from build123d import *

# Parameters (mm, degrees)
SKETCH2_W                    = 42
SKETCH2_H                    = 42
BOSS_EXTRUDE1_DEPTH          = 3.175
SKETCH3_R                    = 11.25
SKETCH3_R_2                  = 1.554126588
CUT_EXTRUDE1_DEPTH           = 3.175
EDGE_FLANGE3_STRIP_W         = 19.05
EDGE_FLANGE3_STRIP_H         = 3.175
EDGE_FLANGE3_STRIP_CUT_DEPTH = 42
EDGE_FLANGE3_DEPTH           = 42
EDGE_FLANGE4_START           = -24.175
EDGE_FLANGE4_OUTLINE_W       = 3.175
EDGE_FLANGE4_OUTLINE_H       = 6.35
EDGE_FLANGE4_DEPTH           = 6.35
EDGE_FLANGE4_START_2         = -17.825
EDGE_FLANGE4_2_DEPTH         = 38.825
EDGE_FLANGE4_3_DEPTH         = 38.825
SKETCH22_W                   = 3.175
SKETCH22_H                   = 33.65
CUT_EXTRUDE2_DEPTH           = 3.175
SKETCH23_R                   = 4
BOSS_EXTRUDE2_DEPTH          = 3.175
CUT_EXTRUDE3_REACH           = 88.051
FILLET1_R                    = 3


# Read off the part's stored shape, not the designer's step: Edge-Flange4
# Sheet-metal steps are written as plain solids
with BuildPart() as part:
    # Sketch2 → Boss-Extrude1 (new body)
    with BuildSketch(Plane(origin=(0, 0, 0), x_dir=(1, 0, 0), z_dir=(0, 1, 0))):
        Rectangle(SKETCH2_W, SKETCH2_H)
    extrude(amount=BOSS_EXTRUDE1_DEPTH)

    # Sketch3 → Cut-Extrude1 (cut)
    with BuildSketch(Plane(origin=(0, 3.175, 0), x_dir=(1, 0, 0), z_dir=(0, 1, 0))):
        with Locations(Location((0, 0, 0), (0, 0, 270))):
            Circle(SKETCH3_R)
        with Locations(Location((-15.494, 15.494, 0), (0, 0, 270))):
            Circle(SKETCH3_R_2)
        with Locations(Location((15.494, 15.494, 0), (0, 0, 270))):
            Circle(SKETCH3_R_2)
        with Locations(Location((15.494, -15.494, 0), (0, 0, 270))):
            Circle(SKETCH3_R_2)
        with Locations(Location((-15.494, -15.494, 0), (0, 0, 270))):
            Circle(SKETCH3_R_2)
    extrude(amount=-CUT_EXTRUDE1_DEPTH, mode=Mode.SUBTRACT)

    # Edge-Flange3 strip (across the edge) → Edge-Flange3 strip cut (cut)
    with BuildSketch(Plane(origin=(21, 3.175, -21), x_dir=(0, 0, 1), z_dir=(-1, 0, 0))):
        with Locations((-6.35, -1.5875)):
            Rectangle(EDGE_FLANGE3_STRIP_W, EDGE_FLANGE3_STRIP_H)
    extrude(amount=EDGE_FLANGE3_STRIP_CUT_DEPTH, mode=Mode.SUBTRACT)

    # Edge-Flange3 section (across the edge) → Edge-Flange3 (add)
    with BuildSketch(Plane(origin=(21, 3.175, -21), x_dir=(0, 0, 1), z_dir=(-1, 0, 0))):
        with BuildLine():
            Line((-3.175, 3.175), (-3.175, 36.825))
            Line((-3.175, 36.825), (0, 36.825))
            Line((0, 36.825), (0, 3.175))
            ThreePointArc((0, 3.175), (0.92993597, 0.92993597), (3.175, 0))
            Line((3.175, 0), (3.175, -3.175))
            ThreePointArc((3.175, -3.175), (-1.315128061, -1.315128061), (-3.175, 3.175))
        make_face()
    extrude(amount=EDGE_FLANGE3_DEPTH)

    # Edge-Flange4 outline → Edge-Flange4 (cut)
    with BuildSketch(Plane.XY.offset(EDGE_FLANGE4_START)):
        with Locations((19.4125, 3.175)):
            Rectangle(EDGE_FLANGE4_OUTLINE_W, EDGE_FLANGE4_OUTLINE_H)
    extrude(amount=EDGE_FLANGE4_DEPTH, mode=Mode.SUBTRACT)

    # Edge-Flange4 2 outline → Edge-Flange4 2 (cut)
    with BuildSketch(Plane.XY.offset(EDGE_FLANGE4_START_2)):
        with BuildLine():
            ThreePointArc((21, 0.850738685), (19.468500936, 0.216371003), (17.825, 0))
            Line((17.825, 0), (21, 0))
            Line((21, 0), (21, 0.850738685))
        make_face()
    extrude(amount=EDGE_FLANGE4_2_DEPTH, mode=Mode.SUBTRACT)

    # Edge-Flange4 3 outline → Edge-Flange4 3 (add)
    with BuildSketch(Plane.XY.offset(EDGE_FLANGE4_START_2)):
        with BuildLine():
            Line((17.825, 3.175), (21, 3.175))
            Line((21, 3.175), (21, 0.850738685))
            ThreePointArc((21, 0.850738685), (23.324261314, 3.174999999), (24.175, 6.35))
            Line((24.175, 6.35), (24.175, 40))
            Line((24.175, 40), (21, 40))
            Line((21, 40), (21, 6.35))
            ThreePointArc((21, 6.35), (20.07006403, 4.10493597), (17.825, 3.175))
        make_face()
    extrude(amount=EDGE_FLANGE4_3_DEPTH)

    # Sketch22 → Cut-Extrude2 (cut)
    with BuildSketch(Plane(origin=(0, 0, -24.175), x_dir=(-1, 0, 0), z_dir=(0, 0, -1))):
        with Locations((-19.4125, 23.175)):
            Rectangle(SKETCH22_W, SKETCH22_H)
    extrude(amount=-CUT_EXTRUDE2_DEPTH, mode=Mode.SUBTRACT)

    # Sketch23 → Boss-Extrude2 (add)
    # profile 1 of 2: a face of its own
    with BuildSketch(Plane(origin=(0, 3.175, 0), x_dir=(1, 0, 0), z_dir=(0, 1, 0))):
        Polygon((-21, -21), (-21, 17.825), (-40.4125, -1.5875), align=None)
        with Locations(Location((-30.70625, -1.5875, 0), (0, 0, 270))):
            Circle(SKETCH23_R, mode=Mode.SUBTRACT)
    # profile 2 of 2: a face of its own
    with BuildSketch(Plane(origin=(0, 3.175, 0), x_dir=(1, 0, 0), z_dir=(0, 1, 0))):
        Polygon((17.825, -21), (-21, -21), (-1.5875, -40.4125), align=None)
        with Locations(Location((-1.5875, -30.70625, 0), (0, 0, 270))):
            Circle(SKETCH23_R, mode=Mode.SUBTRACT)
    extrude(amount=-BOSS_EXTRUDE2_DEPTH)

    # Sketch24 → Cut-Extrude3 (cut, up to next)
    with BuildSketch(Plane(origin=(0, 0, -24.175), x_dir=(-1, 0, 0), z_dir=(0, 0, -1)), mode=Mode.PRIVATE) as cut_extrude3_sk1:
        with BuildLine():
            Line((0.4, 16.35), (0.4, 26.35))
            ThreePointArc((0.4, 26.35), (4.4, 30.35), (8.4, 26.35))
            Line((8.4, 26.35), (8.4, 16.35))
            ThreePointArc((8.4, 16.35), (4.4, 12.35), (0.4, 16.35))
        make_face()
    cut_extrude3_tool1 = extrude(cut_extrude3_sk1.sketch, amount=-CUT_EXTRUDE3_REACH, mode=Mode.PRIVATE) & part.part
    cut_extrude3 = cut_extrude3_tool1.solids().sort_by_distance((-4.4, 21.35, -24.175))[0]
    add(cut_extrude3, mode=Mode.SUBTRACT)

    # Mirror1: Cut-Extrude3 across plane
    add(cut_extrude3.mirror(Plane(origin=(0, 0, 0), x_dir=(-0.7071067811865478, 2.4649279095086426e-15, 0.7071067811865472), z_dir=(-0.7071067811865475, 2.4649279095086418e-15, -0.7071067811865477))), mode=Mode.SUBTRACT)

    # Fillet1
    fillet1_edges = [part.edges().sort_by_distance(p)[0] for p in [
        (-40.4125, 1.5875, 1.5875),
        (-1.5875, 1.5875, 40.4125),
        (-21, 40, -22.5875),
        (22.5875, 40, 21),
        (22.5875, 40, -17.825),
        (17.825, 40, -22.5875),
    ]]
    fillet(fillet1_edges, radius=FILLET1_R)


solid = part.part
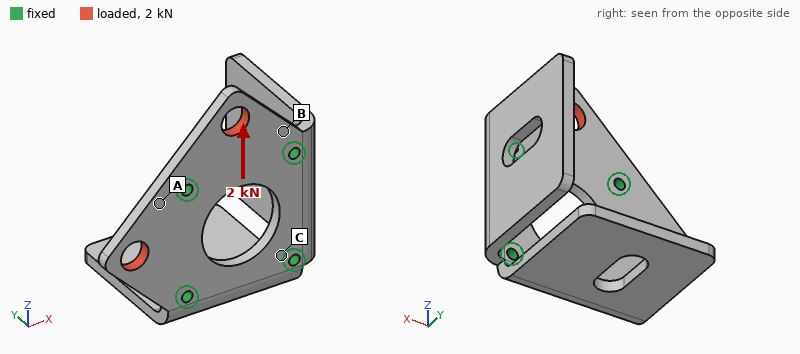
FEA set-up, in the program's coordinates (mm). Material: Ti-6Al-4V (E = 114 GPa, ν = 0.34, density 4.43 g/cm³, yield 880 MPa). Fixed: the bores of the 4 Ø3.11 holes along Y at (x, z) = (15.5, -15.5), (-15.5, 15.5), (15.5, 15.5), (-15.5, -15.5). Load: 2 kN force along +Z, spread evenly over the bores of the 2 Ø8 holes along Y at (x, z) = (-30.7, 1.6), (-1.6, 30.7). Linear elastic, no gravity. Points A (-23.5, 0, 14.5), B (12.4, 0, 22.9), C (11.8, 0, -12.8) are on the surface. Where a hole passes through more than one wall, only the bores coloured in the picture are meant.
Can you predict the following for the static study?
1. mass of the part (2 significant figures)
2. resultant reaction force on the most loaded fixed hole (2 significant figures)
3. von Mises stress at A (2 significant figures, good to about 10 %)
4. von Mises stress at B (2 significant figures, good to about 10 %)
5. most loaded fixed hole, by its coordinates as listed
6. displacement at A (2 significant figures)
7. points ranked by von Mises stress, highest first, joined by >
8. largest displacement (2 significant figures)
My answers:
65 g
1.2 kN
20 MPa
12 MPa
(-15.5, 15.5)
2.3 µm
A > B > C
9.4 µm
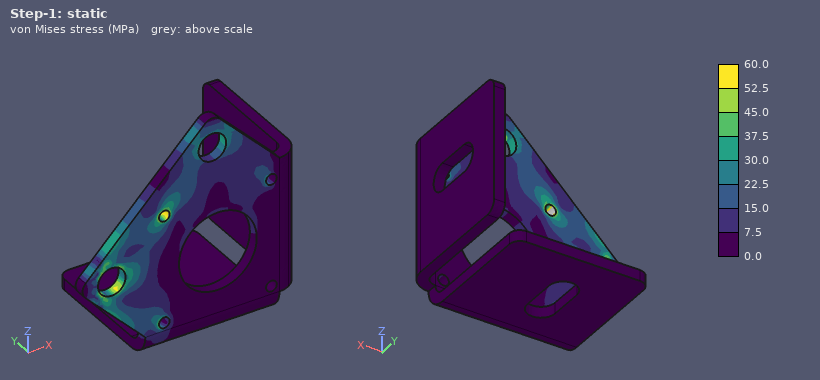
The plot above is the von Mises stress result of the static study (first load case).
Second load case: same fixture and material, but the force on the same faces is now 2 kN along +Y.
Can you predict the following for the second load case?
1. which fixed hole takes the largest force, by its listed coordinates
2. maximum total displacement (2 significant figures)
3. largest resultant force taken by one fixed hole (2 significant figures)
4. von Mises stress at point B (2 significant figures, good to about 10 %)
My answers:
(-15.5, 15.5)
0.36 mm
1.3 kN
190 MPa
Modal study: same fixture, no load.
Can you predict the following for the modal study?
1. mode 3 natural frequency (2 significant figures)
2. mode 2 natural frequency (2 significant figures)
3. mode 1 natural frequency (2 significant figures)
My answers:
3600 Hz
1400 Hz
1400 Hz
